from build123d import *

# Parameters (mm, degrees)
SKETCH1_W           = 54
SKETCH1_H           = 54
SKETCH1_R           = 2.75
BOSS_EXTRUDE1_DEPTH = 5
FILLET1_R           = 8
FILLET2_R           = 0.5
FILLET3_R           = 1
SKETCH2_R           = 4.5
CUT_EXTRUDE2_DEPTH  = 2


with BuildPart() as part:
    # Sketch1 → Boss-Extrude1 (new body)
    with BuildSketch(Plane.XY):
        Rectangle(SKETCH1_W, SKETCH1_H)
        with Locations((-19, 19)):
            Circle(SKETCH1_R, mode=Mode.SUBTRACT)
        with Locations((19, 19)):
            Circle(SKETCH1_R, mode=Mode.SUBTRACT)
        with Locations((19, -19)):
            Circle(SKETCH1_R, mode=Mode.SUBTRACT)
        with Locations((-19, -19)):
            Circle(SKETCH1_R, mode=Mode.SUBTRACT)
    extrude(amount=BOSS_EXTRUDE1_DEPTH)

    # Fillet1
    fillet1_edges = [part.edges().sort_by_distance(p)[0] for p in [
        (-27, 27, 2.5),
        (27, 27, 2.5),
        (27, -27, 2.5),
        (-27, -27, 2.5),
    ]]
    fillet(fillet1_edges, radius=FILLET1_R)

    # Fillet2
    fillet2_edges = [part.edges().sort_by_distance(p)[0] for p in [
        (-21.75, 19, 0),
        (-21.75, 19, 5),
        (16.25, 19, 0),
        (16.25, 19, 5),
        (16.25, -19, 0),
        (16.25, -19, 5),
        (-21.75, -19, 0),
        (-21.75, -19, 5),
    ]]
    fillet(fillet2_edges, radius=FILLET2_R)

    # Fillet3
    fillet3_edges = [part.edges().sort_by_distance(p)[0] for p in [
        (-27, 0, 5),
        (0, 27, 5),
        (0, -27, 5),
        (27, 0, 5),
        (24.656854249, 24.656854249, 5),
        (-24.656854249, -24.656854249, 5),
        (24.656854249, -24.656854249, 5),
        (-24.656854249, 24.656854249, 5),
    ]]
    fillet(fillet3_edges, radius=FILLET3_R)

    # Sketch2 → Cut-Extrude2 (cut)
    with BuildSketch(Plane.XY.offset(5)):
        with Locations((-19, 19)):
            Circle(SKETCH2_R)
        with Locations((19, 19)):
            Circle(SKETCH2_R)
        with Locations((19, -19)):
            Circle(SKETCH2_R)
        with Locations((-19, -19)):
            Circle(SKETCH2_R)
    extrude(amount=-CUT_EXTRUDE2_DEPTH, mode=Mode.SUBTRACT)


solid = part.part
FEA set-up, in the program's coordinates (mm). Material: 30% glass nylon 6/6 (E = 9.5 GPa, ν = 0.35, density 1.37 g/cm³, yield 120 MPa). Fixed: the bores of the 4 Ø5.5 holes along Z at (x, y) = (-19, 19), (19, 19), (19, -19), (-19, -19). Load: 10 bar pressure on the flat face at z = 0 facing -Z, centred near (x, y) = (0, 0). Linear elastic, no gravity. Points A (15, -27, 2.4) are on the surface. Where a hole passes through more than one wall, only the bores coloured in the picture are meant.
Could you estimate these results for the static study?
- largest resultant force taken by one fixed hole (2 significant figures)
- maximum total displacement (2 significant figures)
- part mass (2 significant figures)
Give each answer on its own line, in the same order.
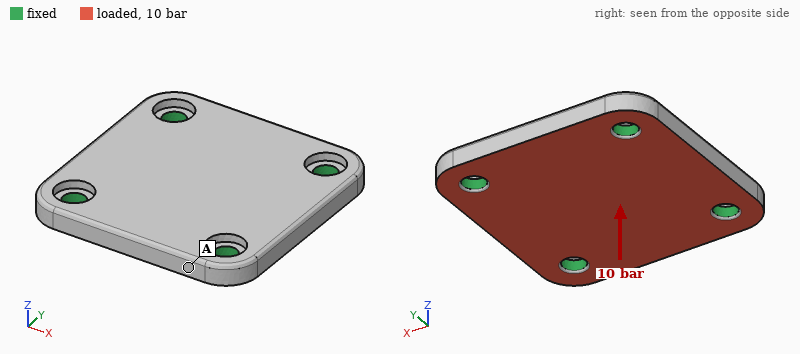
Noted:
750 N
0.17 mm
18 g
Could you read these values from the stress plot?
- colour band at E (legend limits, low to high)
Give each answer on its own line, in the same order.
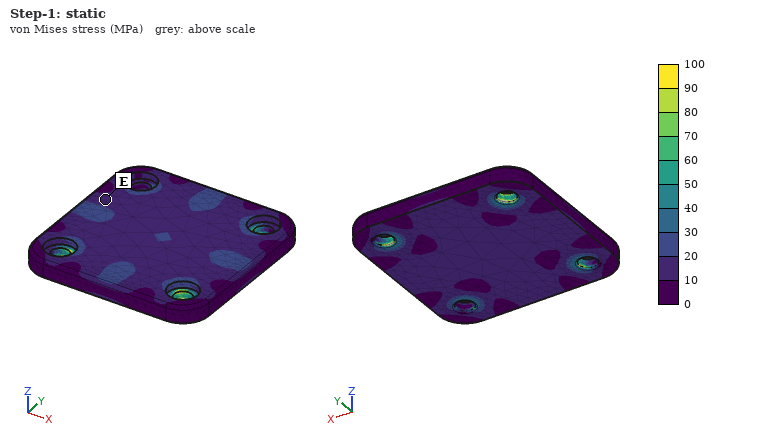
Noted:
10 to 20 MPa
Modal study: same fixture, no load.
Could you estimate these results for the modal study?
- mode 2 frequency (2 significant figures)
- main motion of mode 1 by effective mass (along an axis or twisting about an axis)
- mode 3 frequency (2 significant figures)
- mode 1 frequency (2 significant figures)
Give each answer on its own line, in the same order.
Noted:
7900 Hz
along Z
8000 Hz
5700 Hz
